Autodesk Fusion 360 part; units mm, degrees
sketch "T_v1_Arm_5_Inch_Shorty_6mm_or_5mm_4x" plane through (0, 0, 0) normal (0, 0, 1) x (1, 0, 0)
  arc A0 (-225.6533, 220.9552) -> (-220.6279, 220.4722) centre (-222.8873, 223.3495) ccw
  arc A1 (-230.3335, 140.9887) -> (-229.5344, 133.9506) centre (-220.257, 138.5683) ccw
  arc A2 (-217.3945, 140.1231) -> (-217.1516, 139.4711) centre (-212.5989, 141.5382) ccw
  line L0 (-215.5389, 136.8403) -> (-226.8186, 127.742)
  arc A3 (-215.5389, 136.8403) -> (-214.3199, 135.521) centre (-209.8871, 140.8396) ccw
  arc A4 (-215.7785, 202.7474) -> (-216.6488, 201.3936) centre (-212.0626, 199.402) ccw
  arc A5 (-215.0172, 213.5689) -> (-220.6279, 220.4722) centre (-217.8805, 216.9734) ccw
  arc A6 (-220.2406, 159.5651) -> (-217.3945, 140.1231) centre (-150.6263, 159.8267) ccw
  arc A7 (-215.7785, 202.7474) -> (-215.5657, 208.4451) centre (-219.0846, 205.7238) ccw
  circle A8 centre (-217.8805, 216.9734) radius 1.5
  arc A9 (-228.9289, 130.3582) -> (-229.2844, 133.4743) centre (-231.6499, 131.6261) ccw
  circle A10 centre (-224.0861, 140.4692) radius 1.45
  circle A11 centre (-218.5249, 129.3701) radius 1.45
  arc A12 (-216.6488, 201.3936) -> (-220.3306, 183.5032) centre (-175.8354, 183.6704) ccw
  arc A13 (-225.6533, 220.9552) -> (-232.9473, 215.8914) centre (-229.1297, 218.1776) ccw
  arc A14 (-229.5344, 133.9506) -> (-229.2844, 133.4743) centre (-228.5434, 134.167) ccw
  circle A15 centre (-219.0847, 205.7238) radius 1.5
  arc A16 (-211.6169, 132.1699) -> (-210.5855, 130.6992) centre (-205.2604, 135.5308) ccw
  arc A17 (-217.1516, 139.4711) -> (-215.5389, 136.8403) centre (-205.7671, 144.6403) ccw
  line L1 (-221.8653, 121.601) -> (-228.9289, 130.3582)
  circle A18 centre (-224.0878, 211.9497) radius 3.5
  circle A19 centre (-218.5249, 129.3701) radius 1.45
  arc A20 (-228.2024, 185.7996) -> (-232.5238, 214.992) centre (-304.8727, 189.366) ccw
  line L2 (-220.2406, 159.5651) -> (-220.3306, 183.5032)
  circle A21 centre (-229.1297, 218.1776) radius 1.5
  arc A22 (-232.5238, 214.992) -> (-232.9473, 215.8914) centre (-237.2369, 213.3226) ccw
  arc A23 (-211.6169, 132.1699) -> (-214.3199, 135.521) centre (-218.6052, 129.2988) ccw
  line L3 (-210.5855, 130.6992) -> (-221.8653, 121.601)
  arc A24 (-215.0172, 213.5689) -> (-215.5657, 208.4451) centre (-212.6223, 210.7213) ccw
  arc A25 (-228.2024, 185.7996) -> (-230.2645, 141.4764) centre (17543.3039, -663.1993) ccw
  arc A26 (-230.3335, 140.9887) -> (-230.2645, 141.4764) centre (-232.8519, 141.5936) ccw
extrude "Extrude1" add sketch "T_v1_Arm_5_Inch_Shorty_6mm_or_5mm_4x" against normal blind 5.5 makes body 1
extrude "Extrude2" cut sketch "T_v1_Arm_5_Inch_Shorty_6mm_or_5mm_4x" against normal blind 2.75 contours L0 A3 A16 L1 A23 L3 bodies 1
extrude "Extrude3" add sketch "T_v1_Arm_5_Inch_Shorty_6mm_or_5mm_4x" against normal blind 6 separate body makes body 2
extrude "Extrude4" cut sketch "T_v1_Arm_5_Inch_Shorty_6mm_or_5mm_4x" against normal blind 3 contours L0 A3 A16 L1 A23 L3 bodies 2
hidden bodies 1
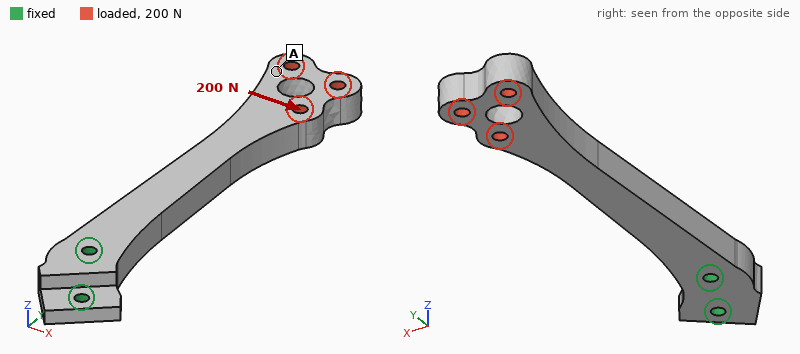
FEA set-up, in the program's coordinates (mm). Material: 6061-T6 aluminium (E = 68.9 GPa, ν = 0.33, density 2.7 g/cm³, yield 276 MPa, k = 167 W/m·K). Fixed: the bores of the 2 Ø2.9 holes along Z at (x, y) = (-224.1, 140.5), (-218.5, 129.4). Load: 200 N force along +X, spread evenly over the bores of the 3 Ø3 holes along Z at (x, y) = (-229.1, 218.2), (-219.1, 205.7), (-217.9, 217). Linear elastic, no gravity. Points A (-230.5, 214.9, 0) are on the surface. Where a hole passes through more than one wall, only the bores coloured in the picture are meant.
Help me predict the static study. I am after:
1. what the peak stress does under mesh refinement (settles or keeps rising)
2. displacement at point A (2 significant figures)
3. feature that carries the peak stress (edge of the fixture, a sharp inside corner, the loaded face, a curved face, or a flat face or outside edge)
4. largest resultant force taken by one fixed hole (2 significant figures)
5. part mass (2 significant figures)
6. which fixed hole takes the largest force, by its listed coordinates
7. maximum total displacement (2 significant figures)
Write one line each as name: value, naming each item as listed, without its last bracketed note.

what the peak stress does under mesh refinement: keeps rising
displacement at point A: 0.99 mm
feature that carries the peak stress: edge of the fixture
largest resultant force taken by one fixed hole: 910 N
part mass: 16 g
which fixed hole takes the largest force, by its listed coordinates: (-224.1, 140.5)
maximum total displacement: 1.1 mm
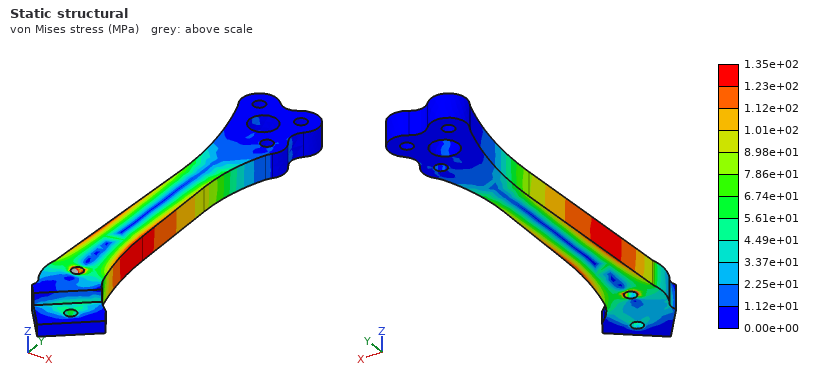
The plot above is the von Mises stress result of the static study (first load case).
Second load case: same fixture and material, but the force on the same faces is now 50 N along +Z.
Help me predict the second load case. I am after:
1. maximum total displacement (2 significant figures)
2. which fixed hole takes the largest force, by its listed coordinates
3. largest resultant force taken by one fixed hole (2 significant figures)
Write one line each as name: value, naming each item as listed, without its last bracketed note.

maximum total displacement: 0.65 mm
which fixed hole takes the largest force, by its listed coordinates: (-224.1, 140.5)
largest resultant force taken by one fixed hole: 110 N
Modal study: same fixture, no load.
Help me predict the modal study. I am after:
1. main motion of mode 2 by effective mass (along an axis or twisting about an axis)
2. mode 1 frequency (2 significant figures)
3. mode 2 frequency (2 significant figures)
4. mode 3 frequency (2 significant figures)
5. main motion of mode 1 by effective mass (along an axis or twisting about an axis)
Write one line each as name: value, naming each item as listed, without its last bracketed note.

main motion of mode 2 by effective mass: along X
mode 1 frequency: 660 Hz
mode 2 frequency: 1000 Hz
mode 3 frequency: 4400 Hz
main motion of mode 1 by effective mass: along Z
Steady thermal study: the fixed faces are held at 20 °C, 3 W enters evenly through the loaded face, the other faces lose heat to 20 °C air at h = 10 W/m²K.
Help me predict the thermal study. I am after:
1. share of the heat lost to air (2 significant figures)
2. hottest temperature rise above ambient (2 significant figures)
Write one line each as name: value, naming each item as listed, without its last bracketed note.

share of the heat lost to air: 12 %
hottest temperature rise above ambient: 21 K
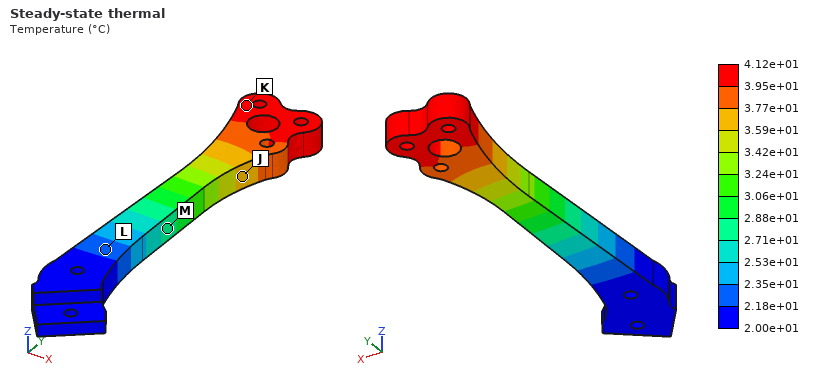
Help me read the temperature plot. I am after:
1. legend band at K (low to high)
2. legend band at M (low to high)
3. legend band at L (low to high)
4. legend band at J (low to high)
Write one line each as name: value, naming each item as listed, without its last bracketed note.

legend band at K: 3.95e+01 to 4.12e+01 °C
legend band at M: 2.71e+01 to 2.88e+01 °C
legend band at L: 2.18e+01 to 2.35e+01 °C
legend band at J: 3.59e+01 to 3.77e+01 °C
